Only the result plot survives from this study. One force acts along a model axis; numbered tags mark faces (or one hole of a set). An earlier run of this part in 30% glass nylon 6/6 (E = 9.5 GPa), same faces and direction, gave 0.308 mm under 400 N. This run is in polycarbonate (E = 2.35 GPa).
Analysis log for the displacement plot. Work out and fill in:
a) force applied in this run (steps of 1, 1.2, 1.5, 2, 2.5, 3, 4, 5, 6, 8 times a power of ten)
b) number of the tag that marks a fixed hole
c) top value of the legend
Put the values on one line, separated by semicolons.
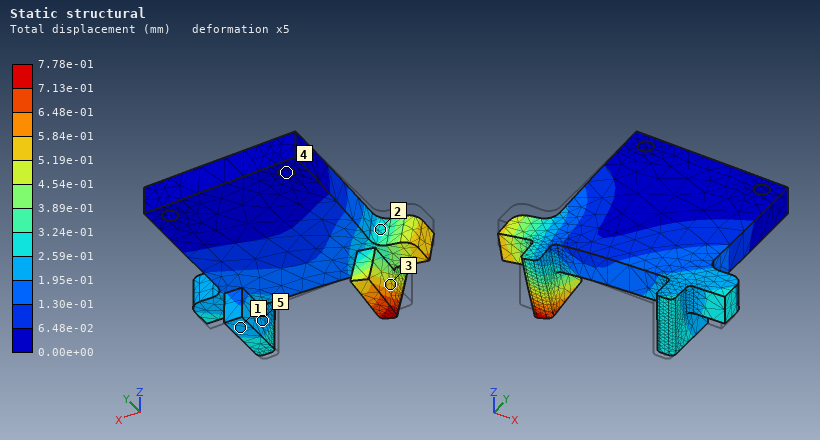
250 N; 4; 7.78e-01 mm
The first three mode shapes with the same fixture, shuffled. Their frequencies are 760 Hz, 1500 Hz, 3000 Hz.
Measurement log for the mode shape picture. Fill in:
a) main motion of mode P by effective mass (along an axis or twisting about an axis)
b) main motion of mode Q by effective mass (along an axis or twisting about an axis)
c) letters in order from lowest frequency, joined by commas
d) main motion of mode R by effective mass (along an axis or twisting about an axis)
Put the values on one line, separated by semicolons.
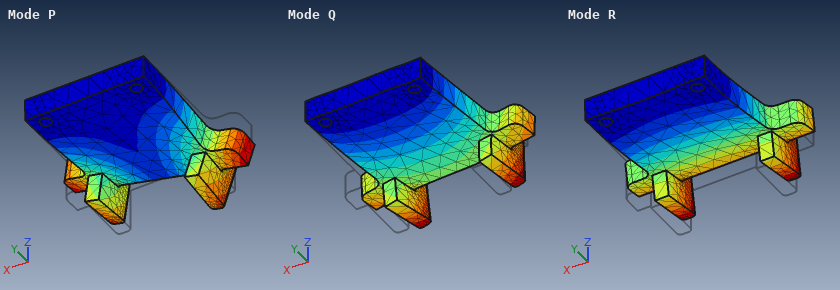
twisting about Y; along X; R, P, Q; along Z
